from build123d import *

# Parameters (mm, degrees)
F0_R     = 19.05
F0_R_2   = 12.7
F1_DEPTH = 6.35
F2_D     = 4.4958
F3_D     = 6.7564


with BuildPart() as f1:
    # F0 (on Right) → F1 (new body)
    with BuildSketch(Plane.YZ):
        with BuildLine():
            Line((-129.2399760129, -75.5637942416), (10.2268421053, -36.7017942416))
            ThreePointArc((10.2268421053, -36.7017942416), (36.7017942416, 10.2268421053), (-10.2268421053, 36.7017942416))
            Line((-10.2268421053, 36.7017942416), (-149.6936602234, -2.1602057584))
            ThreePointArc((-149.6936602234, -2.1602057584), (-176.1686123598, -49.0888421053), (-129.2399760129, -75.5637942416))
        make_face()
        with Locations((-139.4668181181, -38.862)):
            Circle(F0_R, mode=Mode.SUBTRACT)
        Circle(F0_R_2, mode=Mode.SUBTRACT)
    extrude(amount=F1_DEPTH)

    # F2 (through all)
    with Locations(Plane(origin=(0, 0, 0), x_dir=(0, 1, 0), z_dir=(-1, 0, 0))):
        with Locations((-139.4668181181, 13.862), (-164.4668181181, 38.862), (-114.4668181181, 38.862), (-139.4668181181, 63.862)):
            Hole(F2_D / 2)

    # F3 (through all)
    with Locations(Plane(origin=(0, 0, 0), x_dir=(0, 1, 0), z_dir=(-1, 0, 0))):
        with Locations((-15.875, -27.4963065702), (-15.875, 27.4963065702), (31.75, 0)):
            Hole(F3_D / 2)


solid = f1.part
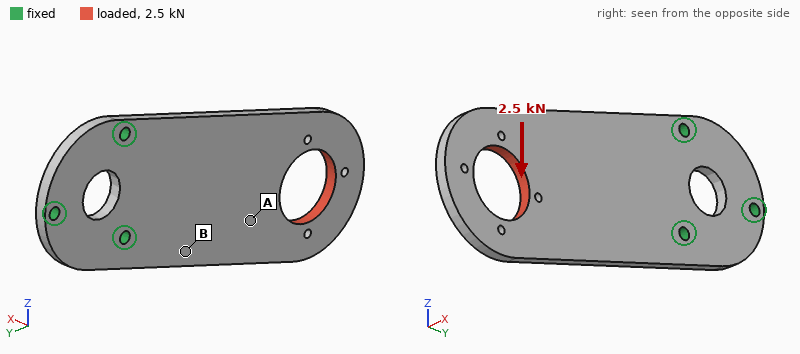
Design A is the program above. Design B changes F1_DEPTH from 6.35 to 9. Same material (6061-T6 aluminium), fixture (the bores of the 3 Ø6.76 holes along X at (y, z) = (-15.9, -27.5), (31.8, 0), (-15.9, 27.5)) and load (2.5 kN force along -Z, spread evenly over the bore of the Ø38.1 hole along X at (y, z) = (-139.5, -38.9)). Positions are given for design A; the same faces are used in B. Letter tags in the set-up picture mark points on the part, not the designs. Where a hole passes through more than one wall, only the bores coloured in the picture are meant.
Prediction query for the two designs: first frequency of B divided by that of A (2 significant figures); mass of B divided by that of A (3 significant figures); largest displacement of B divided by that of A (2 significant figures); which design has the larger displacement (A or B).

1.4
1.42
0.71
A
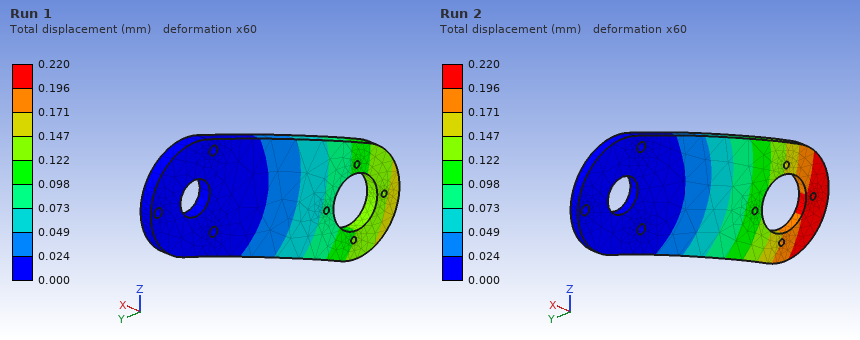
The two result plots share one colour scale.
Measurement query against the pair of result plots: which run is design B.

Run 1
